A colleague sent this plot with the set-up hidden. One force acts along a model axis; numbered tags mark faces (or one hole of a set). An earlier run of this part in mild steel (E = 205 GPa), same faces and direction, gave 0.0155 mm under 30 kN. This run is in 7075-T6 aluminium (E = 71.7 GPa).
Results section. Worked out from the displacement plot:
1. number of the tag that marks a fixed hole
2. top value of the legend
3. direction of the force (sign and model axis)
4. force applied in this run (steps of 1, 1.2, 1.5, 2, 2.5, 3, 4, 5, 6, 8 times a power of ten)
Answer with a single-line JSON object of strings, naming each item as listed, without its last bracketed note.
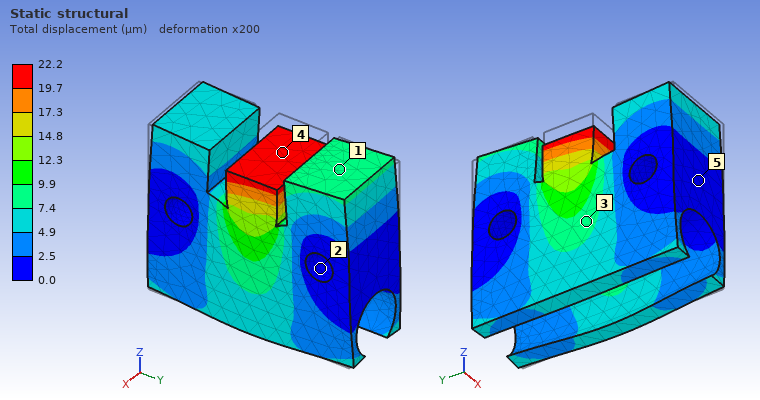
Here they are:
{"number of the tag that marks a fixed hole": "2", "top value of the legend": "22.2 µm", "direction of the force": "-Z", "force applied in this run": "15 kN"}
